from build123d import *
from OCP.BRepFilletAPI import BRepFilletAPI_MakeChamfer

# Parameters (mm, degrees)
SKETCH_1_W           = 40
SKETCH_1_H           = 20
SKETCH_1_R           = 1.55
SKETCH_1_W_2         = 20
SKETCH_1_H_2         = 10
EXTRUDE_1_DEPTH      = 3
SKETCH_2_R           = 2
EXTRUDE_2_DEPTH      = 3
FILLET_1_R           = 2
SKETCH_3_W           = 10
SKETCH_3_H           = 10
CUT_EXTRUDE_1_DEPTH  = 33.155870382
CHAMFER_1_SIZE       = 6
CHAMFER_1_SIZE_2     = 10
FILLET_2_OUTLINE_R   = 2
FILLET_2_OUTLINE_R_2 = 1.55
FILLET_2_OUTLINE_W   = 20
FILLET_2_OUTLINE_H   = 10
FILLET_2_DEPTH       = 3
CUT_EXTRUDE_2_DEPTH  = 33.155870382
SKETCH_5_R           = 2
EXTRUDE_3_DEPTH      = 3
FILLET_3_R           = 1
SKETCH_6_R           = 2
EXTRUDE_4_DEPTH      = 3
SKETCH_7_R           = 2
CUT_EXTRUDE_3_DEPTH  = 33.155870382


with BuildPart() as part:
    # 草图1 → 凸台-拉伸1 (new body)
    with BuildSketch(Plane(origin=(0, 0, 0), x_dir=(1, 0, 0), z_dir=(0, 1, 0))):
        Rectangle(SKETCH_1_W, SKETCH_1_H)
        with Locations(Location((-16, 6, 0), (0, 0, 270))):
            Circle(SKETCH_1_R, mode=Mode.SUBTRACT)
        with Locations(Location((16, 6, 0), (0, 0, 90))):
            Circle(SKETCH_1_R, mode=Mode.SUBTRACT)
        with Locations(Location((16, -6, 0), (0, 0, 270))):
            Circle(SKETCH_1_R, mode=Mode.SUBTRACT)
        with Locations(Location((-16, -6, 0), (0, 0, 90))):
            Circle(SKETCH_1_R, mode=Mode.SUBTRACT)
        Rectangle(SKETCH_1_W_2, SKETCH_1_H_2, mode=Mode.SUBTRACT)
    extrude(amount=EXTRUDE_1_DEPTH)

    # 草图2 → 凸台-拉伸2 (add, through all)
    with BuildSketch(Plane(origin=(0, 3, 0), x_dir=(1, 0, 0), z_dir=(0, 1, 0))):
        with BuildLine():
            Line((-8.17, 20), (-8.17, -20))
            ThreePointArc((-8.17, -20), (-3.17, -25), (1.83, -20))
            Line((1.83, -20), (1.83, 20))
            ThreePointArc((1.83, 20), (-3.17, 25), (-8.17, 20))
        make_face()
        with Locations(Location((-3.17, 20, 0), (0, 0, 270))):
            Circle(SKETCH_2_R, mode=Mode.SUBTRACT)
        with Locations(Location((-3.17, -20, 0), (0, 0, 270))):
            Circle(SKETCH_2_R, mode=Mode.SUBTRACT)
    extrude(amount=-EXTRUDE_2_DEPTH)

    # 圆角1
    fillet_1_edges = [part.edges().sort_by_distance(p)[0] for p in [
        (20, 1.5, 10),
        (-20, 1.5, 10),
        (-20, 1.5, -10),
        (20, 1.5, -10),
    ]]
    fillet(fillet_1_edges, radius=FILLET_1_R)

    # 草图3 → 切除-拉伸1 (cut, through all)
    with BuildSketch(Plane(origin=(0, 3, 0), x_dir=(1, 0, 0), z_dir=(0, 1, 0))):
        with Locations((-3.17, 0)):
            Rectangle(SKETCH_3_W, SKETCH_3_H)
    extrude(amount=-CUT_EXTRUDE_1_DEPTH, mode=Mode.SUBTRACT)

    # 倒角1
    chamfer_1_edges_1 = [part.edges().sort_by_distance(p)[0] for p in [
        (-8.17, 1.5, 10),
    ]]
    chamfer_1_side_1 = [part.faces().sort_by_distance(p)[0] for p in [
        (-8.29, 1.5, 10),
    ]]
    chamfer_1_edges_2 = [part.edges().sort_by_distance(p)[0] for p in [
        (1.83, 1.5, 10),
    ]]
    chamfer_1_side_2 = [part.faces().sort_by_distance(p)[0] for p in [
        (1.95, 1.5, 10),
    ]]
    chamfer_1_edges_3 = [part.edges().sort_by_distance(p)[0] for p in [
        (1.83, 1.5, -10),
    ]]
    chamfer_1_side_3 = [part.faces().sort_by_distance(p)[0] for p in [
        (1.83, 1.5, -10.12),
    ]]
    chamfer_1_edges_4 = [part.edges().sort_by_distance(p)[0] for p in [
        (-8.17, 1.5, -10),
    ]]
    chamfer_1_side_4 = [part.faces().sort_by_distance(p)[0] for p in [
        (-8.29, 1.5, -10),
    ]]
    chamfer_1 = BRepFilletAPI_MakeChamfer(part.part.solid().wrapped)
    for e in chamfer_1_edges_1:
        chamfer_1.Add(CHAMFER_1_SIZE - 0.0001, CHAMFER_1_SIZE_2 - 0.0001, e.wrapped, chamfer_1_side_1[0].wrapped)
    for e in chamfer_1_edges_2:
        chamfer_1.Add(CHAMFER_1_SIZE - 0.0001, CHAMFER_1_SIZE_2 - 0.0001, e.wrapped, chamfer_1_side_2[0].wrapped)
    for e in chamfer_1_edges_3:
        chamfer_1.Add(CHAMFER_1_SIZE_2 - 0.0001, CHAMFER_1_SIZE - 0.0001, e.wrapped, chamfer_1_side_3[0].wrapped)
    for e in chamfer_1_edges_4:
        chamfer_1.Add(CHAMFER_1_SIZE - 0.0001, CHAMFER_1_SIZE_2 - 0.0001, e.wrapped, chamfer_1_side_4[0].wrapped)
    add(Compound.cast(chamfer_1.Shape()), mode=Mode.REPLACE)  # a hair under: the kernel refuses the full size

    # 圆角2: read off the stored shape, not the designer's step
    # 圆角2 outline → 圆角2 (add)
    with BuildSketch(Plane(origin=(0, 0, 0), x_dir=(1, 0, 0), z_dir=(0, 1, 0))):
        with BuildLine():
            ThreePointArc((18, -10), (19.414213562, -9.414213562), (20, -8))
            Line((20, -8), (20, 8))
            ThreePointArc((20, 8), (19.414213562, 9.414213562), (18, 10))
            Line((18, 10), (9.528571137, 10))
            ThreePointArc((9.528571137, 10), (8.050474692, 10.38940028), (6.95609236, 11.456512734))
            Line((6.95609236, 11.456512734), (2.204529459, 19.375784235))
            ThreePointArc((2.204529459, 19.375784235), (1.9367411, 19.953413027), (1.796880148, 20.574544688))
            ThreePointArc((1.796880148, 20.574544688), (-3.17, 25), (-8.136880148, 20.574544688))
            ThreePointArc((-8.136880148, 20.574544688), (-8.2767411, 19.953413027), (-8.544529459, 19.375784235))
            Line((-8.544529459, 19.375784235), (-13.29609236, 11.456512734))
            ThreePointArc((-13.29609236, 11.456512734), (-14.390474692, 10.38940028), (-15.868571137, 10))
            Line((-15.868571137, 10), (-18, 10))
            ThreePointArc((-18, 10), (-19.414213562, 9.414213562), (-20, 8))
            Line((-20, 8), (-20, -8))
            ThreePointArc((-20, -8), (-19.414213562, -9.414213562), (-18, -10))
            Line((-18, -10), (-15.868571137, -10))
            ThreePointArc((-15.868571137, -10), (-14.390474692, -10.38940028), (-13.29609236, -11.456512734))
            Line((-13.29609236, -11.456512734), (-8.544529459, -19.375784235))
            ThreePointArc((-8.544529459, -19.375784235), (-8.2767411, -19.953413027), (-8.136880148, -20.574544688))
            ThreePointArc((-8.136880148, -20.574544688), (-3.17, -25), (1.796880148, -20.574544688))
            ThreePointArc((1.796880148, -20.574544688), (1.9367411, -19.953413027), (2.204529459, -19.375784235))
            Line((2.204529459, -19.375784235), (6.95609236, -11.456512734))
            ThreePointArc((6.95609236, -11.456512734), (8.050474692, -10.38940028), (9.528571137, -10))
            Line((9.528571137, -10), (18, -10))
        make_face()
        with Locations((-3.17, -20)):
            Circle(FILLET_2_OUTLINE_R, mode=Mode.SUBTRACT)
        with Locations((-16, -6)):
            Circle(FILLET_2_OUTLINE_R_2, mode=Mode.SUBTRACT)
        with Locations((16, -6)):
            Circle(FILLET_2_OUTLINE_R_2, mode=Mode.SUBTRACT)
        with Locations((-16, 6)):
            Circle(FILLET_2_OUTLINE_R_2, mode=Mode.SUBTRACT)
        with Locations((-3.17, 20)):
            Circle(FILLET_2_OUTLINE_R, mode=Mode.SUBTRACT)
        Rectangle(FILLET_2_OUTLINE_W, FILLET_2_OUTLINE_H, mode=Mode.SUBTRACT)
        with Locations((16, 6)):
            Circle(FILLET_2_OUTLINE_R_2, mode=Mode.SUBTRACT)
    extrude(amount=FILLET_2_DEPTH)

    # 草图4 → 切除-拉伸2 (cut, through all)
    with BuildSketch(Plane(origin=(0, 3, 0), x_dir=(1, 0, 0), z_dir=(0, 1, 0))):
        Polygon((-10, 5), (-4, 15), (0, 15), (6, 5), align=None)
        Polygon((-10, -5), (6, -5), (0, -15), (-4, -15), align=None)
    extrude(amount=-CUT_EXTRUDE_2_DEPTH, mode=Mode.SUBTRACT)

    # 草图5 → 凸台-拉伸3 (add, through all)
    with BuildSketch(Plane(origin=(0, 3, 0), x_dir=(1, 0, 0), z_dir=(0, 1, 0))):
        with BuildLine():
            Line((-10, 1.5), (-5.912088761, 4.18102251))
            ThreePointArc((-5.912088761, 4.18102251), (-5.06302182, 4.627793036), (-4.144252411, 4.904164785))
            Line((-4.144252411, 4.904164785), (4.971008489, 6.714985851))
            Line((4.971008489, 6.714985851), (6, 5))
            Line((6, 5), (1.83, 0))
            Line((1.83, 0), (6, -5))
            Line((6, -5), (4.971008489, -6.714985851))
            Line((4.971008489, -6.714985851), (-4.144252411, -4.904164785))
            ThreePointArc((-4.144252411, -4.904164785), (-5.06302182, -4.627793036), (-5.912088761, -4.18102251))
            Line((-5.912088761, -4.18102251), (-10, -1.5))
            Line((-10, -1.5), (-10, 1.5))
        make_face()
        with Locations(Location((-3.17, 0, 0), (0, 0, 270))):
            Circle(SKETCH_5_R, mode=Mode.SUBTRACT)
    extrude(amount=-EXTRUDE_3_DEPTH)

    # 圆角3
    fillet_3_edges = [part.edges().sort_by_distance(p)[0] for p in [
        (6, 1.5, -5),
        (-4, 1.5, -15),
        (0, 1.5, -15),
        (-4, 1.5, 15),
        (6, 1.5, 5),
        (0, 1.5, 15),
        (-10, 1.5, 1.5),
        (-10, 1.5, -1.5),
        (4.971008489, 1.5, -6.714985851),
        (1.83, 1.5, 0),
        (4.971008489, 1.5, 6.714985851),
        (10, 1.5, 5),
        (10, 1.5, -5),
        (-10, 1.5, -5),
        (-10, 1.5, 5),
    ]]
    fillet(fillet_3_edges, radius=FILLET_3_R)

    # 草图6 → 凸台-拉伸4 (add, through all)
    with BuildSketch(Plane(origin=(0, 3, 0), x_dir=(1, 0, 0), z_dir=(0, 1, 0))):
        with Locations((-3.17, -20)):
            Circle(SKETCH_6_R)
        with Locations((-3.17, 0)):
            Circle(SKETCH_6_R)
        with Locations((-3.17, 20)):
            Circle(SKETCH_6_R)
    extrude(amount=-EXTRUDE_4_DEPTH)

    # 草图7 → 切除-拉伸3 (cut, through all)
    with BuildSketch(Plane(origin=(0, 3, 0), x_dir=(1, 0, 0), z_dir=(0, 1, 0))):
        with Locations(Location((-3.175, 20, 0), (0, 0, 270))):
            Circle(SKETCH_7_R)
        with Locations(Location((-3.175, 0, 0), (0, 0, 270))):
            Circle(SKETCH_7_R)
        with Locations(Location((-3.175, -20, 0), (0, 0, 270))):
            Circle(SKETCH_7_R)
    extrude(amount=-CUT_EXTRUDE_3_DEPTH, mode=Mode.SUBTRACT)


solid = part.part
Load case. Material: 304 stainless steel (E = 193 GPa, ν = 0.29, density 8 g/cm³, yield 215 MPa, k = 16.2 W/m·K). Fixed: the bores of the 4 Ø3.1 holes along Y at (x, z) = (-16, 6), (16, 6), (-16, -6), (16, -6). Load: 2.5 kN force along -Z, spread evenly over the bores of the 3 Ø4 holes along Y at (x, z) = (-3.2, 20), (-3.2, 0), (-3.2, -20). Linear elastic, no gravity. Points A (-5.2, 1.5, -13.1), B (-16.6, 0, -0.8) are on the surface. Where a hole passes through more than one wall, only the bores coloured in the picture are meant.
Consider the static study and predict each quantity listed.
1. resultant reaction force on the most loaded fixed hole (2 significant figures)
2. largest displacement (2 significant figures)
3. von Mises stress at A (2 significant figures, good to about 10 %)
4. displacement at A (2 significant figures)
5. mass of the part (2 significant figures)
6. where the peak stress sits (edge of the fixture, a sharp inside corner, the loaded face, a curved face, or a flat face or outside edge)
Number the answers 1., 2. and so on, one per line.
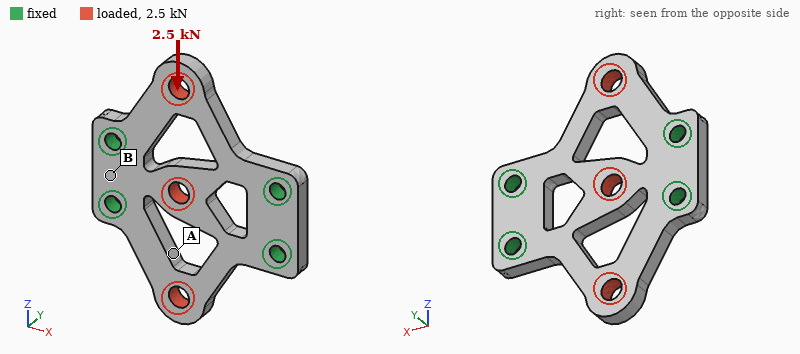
1. 760 N
2. 8.2 µm
3. 44 MPa
4. 4.3 µm
5. 21 g
6. a curved face
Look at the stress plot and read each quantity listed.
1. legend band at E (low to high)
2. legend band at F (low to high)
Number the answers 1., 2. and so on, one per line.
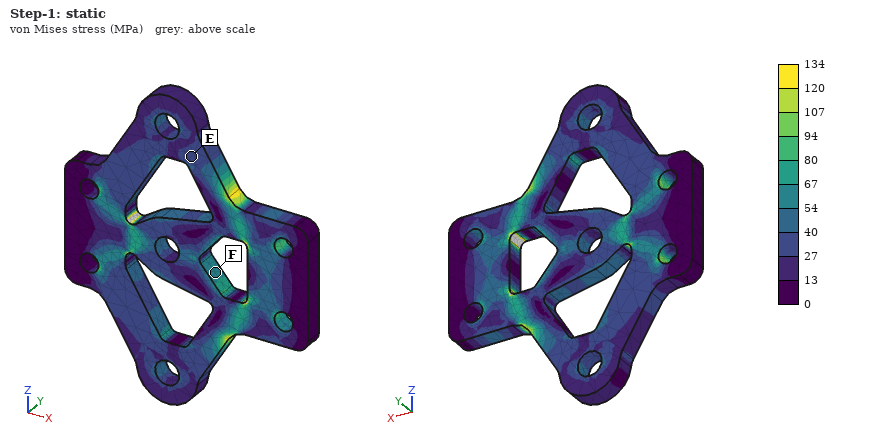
1. 27 to 40 MPa
2. 54 to 67 MPa
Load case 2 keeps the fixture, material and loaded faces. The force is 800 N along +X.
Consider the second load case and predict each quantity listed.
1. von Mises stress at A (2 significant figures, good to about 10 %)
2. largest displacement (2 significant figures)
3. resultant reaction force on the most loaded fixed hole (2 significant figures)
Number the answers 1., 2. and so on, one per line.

1. 14 MPa
2. 3.0 µm
3. 240 N
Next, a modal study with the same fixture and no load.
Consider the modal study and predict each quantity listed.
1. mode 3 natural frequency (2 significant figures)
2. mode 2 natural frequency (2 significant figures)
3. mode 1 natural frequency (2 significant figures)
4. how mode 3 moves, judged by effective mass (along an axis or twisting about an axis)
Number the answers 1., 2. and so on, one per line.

1. 16 kHz
2. 6200 Hz
3. 6100 Hz
4. along Y
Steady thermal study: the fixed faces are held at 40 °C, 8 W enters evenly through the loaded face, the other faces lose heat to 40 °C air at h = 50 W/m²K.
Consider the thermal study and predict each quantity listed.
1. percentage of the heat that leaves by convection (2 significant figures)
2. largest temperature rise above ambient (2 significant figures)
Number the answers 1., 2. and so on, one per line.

1. 42 %
2. 74 K
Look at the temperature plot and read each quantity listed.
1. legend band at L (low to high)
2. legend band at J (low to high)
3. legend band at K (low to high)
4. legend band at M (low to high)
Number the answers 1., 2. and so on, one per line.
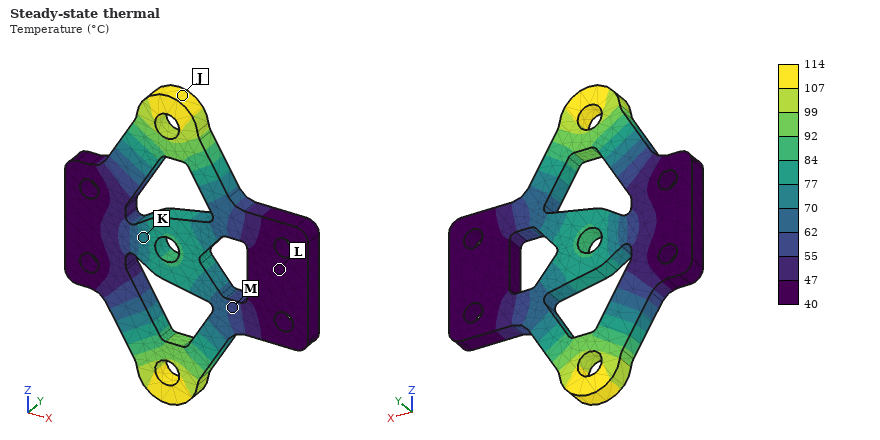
1. 40 to 47 °C
2. 107 to 114 °C
3. 70 to 77 °C
4. 55 to 62 °C
